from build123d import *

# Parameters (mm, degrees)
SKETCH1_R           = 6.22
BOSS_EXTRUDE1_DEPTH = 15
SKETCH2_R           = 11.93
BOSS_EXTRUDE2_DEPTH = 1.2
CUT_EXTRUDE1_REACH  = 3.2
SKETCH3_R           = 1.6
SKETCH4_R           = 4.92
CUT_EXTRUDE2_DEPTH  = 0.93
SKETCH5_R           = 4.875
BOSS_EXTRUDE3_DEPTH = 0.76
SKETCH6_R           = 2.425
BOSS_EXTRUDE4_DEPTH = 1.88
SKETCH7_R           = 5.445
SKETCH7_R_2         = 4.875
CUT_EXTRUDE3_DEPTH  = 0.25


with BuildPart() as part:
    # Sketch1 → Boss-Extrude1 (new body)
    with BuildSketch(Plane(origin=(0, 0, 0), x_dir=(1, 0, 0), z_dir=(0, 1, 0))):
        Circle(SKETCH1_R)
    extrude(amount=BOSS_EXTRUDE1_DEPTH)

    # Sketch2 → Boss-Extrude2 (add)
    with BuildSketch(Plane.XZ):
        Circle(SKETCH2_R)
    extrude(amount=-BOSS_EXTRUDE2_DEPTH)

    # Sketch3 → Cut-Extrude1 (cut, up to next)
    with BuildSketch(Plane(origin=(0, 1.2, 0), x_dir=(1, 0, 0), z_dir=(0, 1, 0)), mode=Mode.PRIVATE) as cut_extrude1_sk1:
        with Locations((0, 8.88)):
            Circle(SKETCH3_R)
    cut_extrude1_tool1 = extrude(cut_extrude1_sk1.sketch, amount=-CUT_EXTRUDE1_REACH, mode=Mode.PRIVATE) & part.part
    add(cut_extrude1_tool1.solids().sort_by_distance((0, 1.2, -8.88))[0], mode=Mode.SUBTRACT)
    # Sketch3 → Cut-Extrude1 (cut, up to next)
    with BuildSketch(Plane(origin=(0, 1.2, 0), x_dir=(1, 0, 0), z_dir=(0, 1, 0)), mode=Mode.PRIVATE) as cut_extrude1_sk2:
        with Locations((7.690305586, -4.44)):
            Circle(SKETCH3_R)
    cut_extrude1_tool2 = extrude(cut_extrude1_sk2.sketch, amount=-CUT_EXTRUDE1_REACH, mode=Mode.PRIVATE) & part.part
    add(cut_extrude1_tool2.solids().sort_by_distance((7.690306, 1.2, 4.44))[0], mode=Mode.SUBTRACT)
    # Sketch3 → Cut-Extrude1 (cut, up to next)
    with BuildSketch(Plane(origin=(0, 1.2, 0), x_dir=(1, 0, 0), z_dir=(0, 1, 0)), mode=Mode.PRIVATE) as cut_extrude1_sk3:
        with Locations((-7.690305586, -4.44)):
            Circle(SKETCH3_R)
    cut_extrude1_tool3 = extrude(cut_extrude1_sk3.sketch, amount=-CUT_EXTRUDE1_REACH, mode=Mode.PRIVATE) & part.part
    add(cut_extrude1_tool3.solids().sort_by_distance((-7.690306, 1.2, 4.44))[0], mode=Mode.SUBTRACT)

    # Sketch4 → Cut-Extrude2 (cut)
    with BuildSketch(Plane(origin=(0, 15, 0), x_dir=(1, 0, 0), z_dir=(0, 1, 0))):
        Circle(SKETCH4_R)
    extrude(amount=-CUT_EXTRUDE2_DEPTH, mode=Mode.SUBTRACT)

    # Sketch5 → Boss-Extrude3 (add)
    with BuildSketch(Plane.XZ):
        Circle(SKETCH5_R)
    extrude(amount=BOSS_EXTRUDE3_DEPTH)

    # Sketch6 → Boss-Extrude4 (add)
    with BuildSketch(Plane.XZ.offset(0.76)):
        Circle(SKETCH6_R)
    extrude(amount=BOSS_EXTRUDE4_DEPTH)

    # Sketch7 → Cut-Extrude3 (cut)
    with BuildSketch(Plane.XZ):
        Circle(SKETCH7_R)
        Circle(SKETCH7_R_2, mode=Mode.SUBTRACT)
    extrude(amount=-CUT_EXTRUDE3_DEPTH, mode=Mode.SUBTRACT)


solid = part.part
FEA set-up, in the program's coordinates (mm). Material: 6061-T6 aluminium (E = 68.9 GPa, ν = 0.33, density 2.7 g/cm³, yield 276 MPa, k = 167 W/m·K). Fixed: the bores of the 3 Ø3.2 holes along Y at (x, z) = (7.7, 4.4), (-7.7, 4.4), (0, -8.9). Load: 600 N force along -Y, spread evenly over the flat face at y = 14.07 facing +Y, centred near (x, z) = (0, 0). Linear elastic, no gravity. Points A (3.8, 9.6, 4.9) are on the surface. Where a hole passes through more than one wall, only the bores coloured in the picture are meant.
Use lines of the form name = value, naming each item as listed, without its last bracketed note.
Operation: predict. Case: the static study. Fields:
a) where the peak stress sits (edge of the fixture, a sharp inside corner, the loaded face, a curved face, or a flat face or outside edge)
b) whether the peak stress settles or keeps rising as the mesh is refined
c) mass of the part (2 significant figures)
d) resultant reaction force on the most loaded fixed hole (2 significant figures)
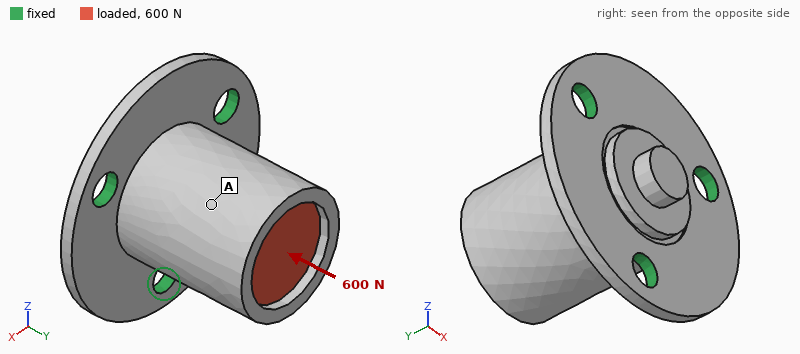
where the peak stress sits = edge of the fixture
whether the peak stress settles or keeps rising as the mesh is refined = keeps rising
mass of the part = 5.9 g
resultant reaction force on the most loaded fixed hole = 220 N
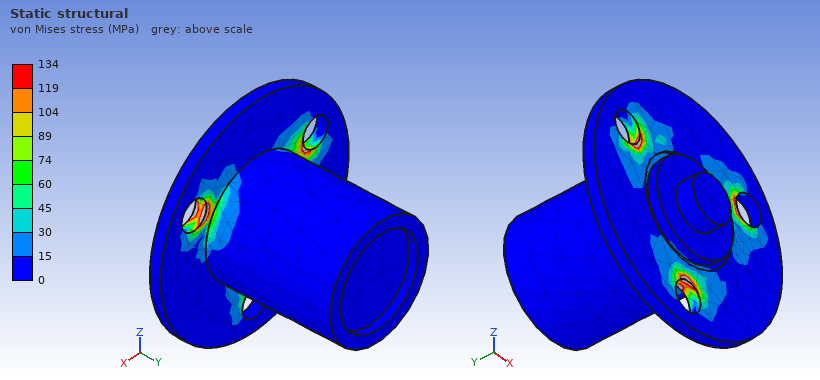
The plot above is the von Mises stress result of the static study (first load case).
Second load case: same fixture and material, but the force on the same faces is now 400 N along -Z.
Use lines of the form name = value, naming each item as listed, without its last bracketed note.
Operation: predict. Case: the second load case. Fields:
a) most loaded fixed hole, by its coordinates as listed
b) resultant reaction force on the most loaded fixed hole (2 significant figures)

most loaded fixed hole, by its coordinates as listed = (0, -8.9)
resultant reaction force on the most loaded fixed hole = 550 N
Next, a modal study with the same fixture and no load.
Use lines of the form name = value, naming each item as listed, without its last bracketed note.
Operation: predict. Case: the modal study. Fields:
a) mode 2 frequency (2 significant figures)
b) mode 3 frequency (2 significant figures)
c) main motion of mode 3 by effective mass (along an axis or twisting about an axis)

mode 2 frequency = 13 kHz
mode 3 frequency = 22 kHz
main motion of mode 3 by effective mass = along Y
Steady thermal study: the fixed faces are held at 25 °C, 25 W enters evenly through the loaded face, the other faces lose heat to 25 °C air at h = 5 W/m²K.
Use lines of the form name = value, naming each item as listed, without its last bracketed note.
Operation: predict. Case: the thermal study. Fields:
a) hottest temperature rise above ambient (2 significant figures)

hottest temperature rise above ambient = 31 K
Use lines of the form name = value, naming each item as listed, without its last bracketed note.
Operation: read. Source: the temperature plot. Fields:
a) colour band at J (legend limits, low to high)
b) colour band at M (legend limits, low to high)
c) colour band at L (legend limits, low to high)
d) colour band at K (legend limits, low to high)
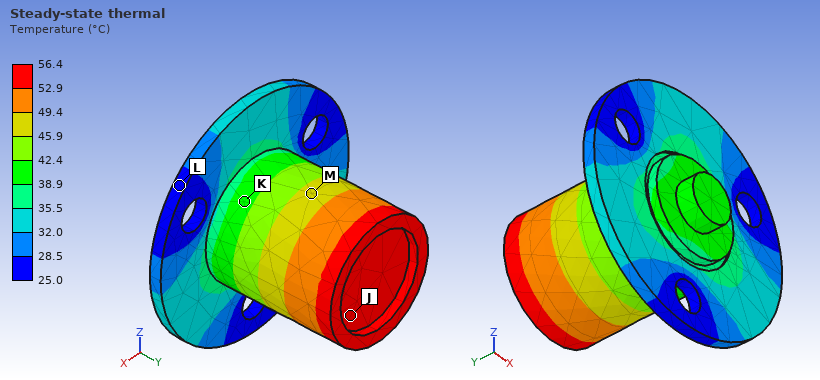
colour band at J = 52.9 to 56.4 °C
colour band at M = 45.9 to 49.4 °C
colour band at L = 25.0 to 28.5 °C
colour band at K = 38.9 to 42.4 °C
